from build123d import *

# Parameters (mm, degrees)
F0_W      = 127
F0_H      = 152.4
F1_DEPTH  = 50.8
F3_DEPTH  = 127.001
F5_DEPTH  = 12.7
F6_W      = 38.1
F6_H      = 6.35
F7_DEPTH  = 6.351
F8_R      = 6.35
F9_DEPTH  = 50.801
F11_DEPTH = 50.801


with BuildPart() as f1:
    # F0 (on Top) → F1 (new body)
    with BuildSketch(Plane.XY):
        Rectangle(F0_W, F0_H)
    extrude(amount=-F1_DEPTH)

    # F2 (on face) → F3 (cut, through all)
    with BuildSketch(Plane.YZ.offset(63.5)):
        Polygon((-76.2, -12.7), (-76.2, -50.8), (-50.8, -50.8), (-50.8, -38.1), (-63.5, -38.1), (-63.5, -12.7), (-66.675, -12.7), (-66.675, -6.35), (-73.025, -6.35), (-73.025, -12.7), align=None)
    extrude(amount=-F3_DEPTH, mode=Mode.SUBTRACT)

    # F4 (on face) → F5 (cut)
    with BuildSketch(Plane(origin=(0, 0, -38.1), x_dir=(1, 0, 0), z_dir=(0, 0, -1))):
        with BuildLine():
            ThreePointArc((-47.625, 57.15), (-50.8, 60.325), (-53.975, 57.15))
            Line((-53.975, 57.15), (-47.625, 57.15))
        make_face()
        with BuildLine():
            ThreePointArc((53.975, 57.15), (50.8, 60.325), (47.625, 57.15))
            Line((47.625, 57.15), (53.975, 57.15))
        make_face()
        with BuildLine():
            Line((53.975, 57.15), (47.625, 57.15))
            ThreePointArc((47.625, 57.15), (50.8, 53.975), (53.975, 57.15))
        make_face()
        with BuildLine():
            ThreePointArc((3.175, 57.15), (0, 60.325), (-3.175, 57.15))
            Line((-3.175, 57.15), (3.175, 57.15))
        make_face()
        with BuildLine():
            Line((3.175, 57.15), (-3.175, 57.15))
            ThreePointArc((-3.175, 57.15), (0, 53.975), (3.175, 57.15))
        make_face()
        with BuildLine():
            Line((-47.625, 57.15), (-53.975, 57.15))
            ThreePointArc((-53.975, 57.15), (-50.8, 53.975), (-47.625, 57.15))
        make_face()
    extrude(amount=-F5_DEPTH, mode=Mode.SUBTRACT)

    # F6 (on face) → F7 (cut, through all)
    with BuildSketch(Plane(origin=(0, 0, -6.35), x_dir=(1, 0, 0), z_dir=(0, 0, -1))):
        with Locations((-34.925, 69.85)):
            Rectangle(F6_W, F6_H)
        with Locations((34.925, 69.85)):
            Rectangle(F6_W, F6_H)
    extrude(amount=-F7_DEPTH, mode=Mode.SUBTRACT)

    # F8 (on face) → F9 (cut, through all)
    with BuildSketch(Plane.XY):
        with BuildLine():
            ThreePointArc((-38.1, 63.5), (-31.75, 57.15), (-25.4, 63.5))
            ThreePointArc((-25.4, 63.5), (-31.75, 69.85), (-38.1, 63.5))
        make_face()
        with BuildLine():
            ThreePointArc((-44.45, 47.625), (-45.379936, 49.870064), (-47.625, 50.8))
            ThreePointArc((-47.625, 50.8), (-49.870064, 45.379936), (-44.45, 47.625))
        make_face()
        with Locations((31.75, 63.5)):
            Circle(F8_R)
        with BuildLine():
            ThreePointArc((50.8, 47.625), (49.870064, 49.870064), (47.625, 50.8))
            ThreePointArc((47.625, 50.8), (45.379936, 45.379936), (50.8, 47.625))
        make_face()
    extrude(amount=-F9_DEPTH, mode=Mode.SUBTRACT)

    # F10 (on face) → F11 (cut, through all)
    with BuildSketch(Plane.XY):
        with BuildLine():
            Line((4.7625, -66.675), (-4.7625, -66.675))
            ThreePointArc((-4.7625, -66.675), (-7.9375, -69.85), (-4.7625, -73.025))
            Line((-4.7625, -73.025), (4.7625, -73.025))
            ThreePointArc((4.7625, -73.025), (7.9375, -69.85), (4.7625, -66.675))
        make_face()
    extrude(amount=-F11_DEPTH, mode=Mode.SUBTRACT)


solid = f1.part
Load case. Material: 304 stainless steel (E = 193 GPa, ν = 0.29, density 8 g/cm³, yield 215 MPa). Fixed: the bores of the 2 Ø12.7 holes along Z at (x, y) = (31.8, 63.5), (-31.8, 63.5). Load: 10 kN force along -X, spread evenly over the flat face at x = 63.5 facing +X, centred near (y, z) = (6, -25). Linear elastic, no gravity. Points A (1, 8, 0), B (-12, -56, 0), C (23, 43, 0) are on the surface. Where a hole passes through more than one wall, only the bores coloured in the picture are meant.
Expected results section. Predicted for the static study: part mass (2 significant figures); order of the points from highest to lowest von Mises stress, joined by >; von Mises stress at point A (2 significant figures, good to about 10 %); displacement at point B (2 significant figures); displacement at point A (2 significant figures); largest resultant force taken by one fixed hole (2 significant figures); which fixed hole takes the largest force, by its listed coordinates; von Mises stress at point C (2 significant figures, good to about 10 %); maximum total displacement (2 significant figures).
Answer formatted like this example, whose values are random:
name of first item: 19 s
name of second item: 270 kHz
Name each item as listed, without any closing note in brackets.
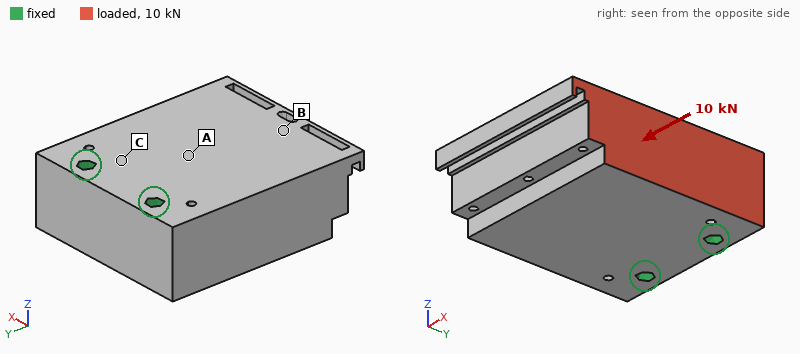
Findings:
part mass: 7.0 kg
order of the points from highest to lowest von Mises stress, joined by >: C > A > B
von Mises stress at point A: 2.8 MPa
displacement at point B: 4.3 µm
displacement at point A: 2.0 µm
largest resultant force taken by one fixed hole: 9.7 kN
which fixed hole takes the largest force, by its listed coordinates: (31.8, 63.5)
von Mises stress at point C: 5.1 MPa
maximum total displacement: 6.0 µm
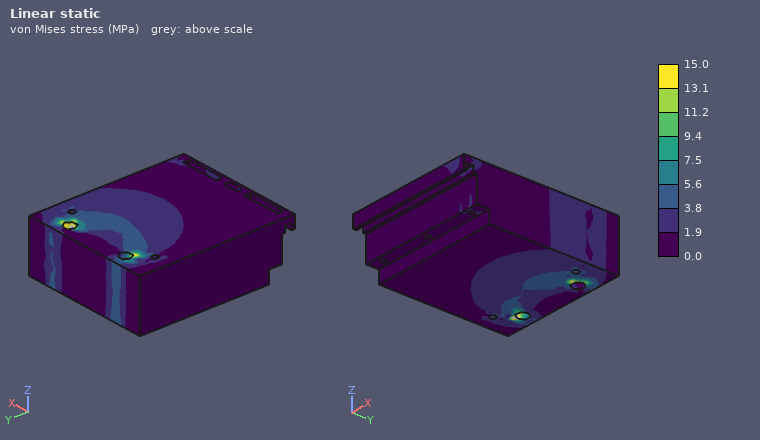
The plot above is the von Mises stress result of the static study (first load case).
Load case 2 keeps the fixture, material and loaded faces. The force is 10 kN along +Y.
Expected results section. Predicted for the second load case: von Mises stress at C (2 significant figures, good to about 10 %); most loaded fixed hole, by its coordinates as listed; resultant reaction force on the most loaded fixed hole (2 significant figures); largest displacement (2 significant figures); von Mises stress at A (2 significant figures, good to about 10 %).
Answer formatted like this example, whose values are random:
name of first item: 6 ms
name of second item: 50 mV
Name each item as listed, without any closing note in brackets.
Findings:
von Mises stress at C: 4.7 MPa
most loaded fixed hole, by its coordinates as listed: (31.8, 63.5)
resultant reaction force on the most loaded fixed hole: 14 kN
largest displacement: 7.0 µm
von Mises stress at A: 1.4 MPa
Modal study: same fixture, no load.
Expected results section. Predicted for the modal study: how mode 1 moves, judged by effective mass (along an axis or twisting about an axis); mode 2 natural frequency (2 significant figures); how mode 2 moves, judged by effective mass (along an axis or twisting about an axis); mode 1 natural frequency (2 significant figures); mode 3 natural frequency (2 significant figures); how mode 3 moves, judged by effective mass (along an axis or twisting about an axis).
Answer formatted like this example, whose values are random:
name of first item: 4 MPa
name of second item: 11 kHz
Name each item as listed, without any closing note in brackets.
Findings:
how mode 1 moves, judged by effective mass: along Z
mode 2 natural frequency: 3200 Hz
how mode 2 moves, judged by effective mass: along X
mode 1 natural frequency: 2000 Hz
mode 3 natural frequency: 4200 Hz
how mode 3 moves, judged by effective mass: twisting about Y
